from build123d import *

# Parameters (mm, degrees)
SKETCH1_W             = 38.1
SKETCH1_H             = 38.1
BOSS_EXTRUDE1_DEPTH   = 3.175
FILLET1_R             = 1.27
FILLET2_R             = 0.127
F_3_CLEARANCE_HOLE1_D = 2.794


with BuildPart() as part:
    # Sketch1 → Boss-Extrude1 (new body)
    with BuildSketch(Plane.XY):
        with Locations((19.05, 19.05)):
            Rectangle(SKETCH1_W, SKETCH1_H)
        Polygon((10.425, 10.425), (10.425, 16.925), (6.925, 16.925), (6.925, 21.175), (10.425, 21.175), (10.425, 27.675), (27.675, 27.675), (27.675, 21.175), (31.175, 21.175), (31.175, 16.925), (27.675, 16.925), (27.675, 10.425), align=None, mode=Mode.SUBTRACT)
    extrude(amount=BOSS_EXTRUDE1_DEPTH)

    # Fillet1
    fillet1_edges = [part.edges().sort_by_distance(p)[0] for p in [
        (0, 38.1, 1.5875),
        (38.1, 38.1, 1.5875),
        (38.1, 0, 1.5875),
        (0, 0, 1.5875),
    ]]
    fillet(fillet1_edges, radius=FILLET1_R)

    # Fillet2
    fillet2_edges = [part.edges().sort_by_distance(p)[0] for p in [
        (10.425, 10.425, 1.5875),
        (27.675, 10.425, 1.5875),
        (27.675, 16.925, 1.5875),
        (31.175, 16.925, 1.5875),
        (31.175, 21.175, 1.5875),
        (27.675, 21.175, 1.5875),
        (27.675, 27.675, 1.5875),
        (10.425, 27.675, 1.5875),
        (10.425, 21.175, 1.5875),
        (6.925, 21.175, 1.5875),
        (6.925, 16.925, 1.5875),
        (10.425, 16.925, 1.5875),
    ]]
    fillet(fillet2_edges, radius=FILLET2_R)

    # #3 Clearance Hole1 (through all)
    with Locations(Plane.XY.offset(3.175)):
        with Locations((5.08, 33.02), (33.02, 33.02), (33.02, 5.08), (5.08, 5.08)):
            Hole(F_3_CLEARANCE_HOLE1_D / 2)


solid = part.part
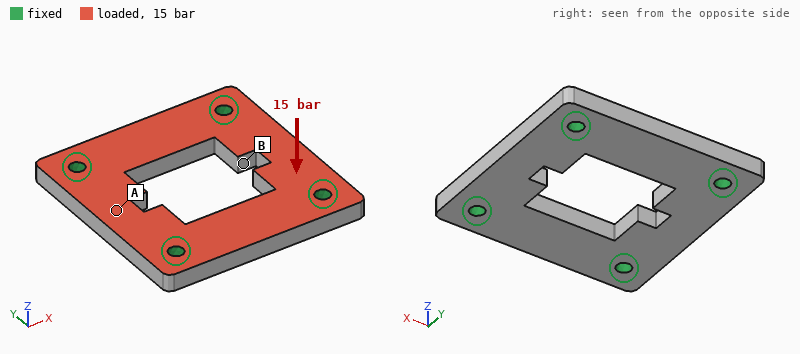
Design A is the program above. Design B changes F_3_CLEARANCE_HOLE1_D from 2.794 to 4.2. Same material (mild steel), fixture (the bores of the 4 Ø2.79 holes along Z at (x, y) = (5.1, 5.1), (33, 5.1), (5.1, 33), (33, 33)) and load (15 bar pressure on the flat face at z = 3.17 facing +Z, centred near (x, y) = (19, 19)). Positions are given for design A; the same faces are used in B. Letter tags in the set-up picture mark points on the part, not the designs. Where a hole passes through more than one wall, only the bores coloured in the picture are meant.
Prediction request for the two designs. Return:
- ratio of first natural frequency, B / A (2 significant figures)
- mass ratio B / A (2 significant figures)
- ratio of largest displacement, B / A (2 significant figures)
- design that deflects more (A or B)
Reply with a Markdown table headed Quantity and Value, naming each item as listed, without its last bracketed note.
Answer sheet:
| Quantity | Value |
|---|---|
| ratio of first natural frequency, B / A | 1.2 |
| mass ratio B / A | 0.97 |
| ratio of largest displacement, B / A | 0.72 |
| design that deflects more | A |
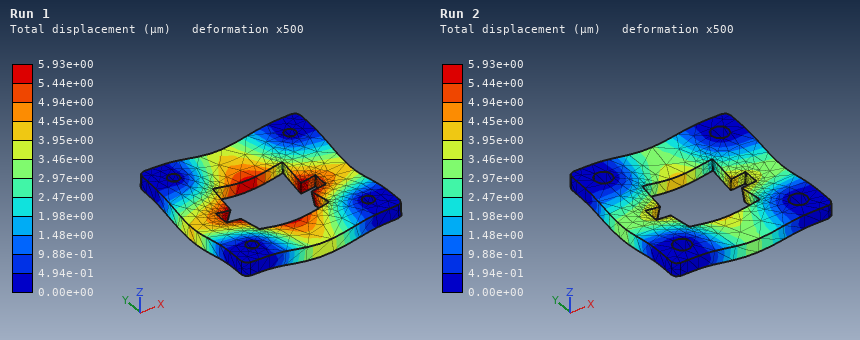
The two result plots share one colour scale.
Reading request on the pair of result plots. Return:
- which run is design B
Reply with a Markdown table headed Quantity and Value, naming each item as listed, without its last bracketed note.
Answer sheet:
| Quantity | Value |
|---|---|
| which run is design B | Run 2 |
